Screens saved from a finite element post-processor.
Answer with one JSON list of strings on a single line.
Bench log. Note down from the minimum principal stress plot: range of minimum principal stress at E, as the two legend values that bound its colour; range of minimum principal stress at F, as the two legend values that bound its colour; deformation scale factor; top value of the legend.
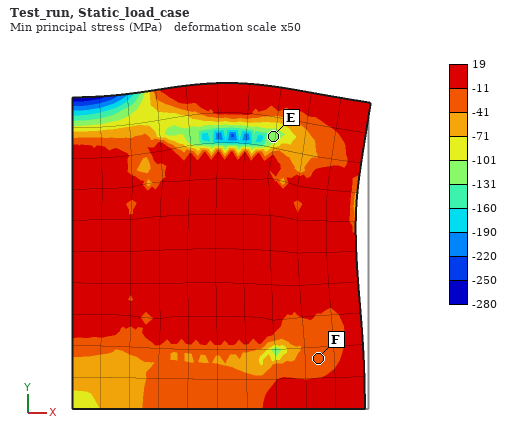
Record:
["-131 to -101 MPa", "-41 to -11 MPa", "50", "19 MPa"]
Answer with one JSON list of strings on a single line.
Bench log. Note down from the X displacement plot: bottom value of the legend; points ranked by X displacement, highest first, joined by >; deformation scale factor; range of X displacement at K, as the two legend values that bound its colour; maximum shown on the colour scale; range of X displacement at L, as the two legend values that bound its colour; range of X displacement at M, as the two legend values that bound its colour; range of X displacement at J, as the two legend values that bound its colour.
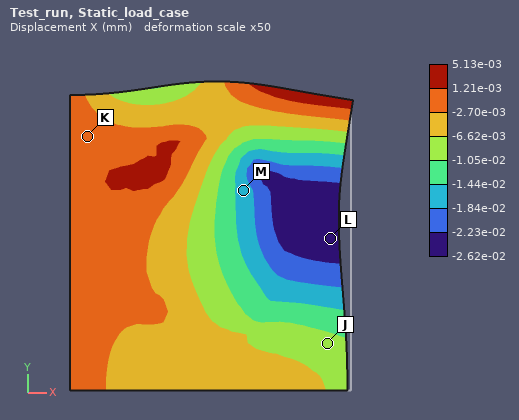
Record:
["-2.62e-02 mm", "K > J > M > L", "50", "-2.70e-03 to 1.21e-03 mm", "5.13e-03 mm", "-2.62e-02 to -2.23e-02 mm", "-1.84e-02 to -1.44e-02 mm", "-1.05e-02 to -6.62e-03 mm"]
